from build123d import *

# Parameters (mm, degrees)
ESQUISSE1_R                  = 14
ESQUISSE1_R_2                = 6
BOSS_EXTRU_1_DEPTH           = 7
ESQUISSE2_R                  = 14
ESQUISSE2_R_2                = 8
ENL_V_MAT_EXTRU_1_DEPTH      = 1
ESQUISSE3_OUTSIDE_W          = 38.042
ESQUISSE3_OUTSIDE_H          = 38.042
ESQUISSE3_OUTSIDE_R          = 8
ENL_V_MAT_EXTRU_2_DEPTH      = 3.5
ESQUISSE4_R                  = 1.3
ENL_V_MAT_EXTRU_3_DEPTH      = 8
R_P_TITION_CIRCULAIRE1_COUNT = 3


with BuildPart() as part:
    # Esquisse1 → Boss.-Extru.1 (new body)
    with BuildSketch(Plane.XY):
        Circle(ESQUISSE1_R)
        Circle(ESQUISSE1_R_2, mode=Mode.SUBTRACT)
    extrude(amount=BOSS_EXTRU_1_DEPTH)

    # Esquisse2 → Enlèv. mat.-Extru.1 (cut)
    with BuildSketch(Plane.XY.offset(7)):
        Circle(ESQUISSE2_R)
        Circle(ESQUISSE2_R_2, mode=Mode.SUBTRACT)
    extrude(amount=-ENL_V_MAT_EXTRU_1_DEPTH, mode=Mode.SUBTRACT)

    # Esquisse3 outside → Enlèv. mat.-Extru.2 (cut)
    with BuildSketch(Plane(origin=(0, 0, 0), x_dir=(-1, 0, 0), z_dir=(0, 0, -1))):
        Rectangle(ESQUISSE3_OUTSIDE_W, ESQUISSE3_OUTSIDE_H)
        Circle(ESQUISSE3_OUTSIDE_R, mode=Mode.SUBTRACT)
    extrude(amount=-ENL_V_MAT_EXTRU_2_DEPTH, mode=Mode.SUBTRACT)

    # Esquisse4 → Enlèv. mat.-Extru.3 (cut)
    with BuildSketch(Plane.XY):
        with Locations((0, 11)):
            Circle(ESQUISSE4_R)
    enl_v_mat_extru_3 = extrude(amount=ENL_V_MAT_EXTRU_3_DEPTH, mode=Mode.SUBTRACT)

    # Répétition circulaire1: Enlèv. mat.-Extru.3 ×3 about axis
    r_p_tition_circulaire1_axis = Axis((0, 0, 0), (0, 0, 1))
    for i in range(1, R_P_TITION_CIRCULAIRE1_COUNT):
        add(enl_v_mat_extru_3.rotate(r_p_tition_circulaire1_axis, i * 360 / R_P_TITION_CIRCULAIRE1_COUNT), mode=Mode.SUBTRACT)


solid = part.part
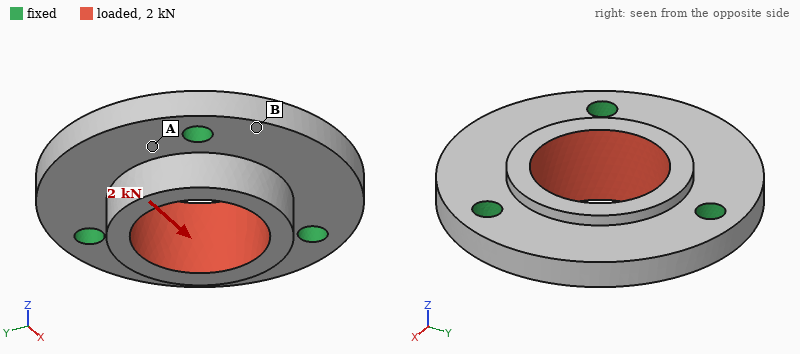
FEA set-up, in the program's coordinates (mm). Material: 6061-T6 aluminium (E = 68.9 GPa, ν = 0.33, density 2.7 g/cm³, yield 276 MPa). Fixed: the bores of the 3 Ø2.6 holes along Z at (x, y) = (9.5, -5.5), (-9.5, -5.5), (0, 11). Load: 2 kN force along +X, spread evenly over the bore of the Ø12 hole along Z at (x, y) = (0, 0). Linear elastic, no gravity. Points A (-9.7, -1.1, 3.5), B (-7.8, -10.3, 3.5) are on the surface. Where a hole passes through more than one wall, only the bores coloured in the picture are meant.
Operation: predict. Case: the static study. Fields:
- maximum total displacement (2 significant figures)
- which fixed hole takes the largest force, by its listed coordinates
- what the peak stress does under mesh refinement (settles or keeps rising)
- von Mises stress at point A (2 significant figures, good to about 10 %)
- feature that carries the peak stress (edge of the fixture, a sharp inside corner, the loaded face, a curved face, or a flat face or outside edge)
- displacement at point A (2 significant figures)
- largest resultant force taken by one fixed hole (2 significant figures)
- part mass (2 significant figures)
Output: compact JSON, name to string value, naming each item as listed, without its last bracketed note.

{"maximum total displacement": "11 µm", "which fixed hole takes the largest force, by its listed coordinates": "(0, 11)", "what the peak stress does under mesh refinement": "keeps rising", "von Mises stress at point A": "26 MPa", "feature that carries the peak stress": "edge of the fixture", "displacement at point A": "3.6 µm", "largest resultant force taken by one fixed hole": "770 N", "part mass": "4.4 g"}
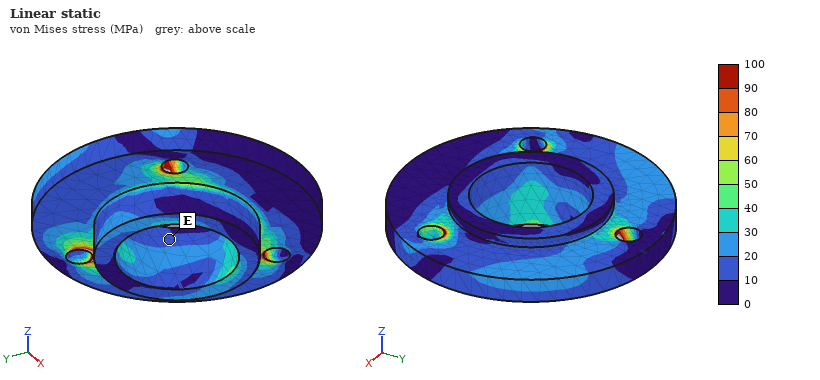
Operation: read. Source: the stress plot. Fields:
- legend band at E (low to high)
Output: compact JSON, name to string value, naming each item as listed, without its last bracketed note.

{"legend band at E": "10 to 20 MPa"}
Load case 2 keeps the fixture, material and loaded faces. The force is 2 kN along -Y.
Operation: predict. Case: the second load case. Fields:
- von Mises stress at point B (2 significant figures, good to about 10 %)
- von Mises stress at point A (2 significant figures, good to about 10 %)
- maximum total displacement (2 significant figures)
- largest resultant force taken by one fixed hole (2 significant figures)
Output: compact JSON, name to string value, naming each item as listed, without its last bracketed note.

{"von Mises stress at point B": "21 MPa", "von Mises stress at point A": "29 MPa", "maximum total displacement": "12 µm", "largest resultant force taken by one fixed hole": "730 N"}
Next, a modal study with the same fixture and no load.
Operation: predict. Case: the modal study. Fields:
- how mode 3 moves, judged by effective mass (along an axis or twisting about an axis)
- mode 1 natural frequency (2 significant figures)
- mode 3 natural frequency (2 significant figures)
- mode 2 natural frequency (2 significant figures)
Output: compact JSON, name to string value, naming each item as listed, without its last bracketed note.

{"how mode 3 moves, judged by effective mass": "along Z", "mode 1 natural frequency": "24 kHz", "mode 3 natural frequency": "30 kHz", "mode 2 natural frequency": "24 kHz"}
